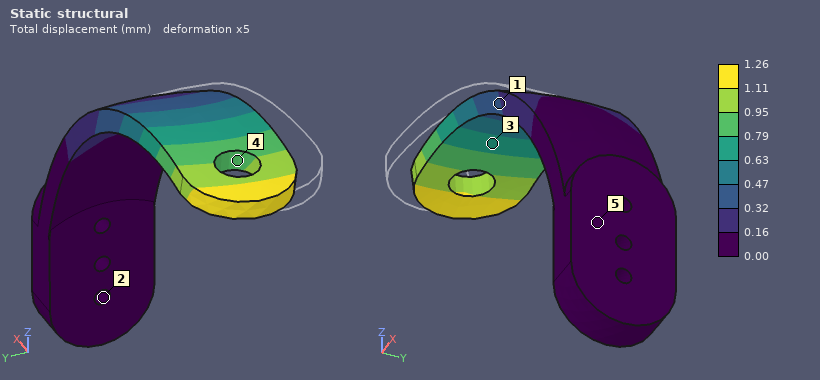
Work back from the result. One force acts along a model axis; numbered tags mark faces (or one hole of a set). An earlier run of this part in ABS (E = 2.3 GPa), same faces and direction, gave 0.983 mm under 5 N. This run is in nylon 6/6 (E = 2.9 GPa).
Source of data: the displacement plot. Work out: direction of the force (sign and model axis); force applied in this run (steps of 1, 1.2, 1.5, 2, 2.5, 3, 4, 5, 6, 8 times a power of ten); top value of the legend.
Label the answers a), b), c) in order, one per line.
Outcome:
a) +Y
b) 8 N
c) 1.26 mm
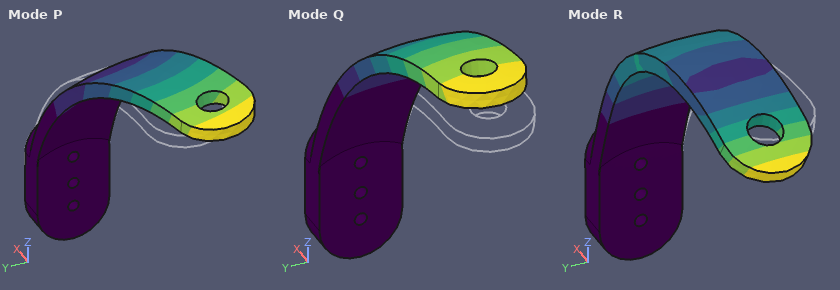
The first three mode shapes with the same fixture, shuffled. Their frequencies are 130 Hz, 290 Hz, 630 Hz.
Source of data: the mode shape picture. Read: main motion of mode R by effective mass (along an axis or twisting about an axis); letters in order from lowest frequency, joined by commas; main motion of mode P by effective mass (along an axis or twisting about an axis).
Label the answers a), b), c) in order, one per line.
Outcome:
a) along X
b) Q, P, R
c) along Y
